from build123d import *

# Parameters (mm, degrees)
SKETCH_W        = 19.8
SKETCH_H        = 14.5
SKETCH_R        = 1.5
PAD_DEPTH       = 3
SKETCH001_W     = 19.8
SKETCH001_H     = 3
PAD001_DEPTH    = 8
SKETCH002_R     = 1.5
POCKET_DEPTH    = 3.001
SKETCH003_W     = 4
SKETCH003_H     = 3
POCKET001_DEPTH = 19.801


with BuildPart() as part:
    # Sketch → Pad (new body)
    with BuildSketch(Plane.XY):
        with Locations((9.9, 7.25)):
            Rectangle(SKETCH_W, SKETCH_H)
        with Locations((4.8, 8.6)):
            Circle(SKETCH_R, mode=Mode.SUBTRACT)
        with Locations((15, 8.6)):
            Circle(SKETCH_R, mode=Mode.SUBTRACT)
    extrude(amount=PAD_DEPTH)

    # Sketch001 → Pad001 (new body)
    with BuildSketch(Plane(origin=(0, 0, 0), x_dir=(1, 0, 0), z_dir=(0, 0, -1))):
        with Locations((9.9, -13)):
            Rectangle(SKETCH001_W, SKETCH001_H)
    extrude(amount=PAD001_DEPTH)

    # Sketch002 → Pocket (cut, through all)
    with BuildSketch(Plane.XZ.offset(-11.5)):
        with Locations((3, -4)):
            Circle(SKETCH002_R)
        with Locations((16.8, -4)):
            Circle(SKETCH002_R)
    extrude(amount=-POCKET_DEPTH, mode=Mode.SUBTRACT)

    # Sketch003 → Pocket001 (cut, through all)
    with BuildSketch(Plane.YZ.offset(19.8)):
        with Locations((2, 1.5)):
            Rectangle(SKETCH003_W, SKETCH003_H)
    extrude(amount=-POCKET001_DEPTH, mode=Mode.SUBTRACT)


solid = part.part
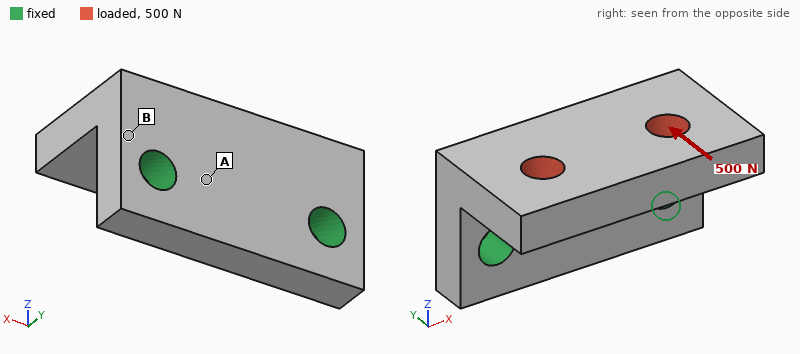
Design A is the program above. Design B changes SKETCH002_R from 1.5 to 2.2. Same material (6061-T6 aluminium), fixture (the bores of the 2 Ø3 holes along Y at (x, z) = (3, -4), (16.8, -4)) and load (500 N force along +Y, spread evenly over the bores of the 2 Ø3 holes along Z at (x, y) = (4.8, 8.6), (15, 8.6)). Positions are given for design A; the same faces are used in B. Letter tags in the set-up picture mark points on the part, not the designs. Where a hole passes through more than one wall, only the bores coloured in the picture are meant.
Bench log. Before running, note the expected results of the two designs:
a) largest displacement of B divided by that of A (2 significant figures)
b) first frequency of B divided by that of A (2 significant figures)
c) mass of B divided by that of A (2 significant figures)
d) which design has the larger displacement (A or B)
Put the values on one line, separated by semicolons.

0.68; 1.1; 0.95; A
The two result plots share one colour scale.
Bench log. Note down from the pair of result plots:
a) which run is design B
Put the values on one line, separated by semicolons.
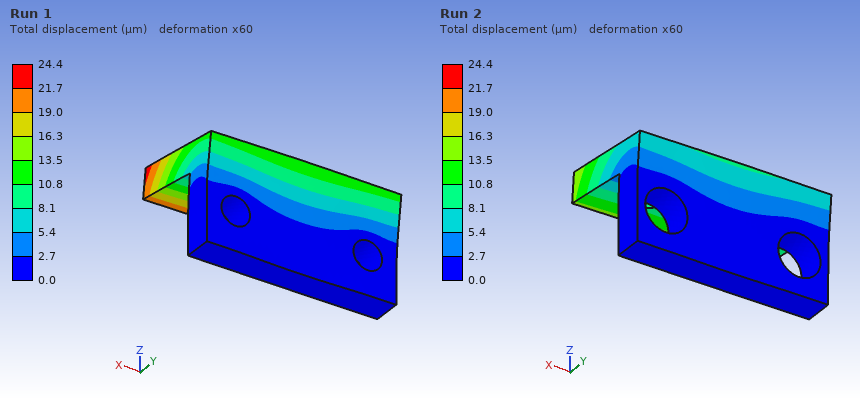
Run 2
